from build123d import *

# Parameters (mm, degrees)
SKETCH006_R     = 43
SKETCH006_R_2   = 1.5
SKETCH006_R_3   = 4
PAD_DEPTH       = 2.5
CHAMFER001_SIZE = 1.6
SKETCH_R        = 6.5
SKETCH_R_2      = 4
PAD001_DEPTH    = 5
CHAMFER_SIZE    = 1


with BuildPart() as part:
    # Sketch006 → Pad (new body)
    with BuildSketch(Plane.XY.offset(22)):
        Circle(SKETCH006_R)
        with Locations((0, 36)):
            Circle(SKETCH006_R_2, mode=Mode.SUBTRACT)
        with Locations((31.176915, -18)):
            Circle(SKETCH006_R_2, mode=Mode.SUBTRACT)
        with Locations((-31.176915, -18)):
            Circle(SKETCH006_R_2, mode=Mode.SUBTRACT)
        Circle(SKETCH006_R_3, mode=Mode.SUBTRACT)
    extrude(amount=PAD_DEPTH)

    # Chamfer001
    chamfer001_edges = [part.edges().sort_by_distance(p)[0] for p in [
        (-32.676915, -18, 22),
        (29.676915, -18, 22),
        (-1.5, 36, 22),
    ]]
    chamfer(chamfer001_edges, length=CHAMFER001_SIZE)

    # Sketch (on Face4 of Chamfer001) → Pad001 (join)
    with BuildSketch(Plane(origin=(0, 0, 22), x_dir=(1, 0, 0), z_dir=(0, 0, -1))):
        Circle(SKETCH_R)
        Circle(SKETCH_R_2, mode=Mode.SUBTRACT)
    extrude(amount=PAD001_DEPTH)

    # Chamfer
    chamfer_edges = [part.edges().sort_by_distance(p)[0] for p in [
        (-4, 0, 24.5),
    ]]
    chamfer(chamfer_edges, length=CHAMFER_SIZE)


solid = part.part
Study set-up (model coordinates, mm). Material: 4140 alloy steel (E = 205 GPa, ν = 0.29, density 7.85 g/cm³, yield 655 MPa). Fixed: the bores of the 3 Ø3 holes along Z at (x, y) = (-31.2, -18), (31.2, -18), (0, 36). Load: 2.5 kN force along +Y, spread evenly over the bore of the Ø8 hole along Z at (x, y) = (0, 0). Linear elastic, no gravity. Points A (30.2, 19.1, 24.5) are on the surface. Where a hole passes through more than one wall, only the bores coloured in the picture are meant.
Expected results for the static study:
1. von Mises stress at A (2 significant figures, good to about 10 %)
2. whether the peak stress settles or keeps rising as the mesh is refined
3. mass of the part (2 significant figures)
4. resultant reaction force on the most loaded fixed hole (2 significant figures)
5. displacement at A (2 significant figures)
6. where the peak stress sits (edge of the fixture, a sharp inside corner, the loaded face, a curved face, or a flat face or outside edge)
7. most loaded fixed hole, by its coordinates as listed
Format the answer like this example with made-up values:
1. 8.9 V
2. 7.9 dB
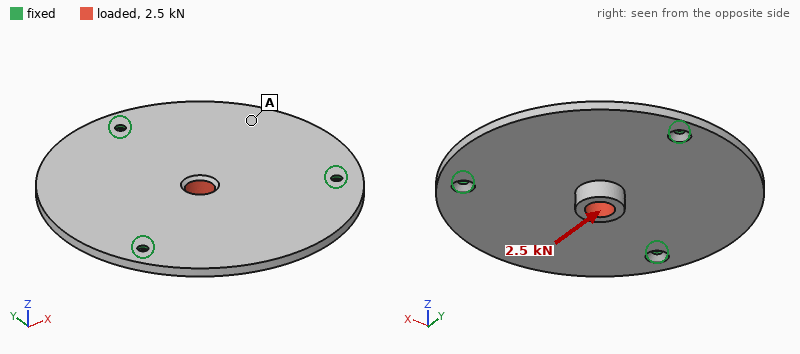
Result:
1. 16 MPa
2. keeps rising
3. 120 g
4. 1.2 kN
5. 22 µm
6. edge of the fixture
7. (0, 36)
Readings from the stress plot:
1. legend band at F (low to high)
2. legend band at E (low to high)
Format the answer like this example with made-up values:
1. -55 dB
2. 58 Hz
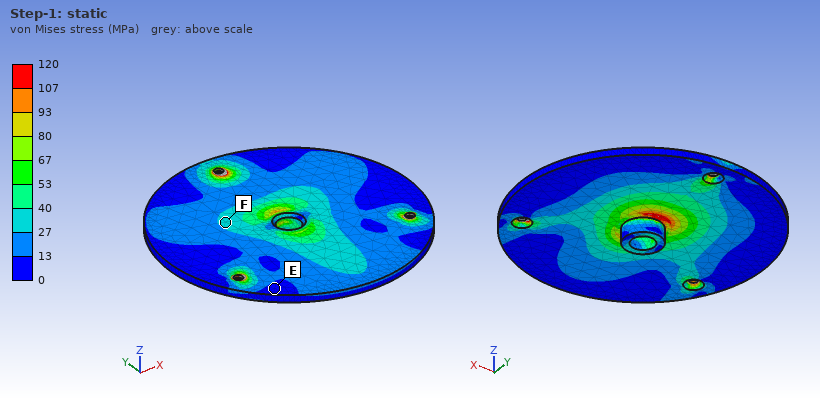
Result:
1. 27 to 40 MPa
2. 0 to 13 MPa
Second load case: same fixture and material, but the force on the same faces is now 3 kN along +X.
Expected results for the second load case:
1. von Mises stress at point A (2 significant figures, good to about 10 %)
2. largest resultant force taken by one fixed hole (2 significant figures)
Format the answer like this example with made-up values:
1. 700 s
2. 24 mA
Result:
1. 28 MPa
2. 1.2 kN
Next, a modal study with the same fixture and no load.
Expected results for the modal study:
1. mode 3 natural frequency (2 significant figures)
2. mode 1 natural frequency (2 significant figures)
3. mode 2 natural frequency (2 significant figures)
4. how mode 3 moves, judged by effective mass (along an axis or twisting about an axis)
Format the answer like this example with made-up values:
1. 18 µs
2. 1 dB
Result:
1. 2200 Hz
2. 1800 Hz
3. 1800 Hz
4. along Z
